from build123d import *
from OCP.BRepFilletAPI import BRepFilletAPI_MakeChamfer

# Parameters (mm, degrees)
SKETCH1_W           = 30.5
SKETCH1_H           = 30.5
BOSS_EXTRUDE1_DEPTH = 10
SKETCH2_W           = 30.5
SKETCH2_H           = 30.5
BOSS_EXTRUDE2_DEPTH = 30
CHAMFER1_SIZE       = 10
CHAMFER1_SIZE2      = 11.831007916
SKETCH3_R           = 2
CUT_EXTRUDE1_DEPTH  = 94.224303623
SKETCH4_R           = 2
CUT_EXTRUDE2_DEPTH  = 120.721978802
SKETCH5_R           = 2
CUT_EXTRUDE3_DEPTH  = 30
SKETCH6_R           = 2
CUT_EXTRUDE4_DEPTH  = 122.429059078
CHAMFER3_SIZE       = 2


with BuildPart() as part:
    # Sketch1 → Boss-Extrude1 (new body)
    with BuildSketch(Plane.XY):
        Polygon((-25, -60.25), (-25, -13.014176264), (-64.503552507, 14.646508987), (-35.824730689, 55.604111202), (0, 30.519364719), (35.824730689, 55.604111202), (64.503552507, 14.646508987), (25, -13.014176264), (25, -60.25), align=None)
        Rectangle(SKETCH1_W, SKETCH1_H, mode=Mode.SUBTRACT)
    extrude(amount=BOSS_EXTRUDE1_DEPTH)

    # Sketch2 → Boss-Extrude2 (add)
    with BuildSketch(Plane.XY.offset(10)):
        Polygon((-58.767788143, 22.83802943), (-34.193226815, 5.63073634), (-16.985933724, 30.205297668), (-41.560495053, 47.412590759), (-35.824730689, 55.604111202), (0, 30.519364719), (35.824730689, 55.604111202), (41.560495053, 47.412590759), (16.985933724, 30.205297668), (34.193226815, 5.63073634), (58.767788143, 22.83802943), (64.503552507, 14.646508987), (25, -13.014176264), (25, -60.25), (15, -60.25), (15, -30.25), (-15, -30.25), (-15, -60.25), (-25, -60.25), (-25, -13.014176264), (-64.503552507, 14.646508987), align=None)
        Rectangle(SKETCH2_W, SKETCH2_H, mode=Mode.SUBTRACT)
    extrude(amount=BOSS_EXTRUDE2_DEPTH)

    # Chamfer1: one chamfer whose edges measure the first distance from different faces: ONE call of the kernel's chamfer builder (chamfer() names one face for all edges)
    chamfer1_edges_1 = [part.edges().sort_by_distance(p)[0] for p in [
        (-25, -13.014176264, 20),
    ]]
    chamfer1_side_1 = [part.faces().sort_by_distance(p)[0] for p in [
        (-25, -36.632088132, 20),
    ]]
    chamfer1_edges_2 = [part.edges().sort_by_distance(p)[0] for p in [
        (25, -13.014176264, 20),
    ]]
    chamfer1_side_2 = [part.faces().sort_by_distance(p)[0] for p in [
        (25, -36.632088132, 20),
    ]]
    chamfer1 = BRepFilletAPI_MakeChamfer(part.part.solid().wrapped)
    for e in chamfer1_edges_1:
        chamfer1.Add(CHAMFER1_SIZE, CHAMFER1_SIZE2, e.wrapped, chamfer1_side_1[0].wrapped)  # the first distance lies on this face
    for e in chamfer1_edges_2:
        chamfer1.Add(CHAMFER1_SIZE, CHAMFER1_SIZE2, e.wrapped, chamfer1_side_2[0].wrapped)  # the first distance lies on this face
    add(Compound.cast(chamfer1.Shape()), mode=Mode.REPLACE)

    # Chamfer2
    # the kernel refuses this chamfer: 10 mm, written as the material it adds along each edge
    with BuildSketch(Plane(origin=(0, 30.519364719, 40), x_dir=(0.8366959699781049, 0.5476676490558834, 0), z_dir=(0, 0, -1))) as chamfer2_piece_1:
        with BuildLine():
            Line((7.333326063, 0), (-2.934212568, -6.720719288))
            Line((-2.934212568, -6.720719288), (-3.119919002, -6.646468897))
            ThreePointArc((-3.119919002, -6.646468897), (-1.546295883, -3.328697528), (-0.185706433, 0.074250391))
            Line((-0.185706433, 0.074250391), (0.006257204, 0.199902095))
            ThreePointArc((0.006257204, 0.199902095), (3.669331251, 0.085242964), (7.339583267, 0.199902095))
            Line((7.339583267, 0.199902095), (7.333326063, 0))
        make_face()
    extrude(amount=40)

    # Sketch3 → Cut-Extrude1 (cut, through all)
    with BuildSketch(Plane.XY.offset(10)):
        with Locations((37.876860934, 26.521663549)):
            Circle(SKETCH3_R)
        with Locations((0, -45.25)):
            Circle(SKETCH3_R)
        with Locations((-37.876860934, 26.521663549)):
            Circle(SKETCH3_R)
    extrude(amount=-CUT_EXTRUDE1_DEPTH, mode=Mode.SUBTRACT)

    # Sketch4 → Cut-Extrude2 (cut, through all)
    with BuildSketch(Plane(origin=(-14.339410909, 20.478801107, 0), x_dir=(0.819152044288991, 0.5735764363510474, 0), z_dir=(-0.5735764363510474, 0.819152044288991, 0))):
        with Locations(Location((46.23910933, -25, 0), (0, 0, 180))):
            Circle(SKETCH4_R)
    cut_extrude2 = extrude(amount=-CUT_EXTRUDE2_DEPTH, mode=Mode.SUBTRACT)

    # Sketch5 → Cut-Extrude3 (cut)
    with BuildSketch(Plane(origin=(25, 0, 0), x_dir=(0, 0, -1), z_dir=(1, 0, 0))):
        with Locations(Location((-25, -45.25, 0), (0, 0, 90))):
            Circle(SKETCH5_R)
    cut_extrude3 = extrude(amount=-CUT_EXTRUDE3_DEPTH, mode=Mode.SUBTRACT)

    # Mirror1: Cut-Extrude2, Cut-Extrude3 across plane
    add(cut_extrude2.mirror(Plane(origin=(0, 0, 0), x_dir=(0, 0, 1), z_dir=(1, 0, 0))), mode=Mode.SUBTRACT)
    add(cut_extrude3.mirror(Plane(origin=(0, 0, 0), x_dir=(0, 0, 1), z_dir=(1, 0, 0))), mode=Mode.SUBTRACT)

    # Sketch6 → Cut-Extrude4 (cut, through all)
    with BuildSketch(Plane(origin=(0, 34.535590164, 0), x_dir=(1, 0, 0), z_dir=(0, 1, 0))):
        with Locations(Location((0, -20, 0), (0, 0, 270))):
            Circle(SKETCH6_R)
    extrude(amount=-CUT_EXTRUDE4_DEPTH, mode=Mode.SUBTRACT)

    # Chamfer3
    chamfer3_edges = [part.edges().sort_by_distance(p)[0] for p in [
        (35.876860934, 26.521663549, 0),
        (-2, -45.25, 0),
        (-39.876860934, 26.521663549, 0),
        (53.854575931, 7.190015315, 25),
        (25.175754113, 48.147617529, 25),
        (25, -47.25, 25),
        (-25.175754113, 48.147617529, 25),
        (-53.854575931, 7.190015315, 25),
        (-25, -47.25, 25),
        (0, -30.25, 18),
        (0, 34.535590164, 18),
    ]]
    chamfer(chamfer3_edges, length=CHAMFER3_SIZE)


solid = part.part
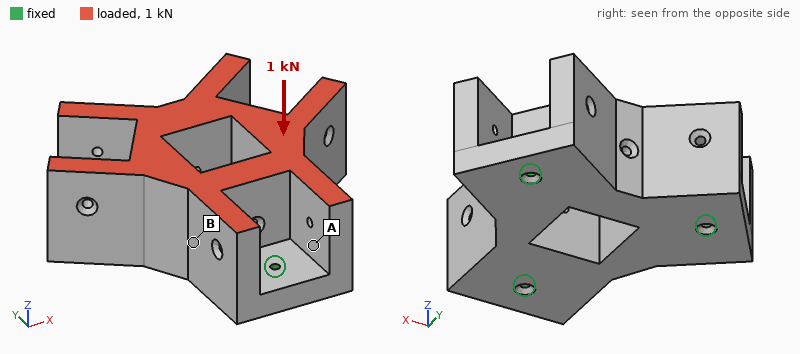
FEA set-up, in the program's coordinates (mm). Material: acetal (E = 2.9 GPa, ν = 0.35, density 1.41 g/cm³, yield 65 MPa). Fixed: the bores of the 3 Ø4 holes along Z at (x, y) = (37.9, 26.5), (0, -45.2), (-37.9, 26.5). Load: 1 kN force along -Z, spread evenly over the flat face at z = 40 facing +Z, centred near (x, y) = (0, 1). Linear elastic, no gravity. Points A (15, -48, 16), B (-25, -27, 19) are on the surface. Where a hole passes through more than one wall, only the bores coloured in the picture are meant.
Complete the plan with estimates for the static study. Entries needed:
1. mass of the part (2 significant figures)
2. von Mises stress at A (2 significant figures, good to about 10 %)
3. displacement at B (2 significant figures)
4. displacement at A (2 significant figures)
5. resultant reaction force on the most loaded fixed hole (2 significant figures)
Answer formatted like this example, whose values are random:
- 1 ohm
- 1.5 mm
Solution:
- 290 g
- 1.2 MPa
- 39 µm
- 32 µm
- 360 N
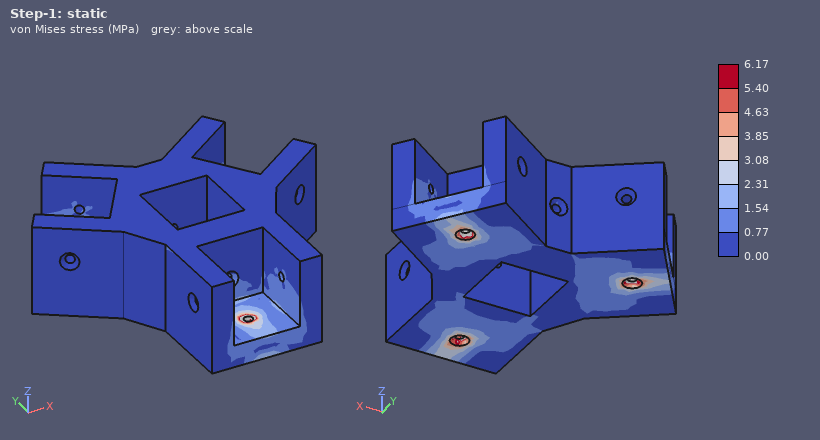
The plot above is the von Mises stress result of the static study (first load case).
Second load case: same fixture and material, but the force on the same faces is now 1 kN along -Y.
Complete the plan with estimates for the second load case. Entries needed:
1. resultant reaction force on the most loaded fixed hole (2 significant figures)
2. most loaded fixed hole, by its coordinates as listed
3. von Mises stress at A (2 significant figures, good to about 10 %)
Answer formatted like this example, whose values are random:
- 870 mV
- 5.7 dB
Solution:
- 630 N
- (0, -45.2)
- 1.7 MPa
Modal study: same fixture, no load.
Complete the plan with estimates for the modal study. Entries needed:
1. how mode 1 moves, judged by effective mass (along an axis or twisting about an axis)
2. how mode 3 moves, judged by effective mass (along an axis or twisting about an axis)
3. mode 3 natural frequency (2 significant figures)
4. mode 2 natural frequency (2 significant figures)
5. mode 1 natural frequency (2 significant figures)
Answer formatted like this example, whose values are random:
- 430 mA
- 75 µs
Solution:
- along X
- along Z
- 1600 Hz
- 1500 Hz
- 1400 Hz
